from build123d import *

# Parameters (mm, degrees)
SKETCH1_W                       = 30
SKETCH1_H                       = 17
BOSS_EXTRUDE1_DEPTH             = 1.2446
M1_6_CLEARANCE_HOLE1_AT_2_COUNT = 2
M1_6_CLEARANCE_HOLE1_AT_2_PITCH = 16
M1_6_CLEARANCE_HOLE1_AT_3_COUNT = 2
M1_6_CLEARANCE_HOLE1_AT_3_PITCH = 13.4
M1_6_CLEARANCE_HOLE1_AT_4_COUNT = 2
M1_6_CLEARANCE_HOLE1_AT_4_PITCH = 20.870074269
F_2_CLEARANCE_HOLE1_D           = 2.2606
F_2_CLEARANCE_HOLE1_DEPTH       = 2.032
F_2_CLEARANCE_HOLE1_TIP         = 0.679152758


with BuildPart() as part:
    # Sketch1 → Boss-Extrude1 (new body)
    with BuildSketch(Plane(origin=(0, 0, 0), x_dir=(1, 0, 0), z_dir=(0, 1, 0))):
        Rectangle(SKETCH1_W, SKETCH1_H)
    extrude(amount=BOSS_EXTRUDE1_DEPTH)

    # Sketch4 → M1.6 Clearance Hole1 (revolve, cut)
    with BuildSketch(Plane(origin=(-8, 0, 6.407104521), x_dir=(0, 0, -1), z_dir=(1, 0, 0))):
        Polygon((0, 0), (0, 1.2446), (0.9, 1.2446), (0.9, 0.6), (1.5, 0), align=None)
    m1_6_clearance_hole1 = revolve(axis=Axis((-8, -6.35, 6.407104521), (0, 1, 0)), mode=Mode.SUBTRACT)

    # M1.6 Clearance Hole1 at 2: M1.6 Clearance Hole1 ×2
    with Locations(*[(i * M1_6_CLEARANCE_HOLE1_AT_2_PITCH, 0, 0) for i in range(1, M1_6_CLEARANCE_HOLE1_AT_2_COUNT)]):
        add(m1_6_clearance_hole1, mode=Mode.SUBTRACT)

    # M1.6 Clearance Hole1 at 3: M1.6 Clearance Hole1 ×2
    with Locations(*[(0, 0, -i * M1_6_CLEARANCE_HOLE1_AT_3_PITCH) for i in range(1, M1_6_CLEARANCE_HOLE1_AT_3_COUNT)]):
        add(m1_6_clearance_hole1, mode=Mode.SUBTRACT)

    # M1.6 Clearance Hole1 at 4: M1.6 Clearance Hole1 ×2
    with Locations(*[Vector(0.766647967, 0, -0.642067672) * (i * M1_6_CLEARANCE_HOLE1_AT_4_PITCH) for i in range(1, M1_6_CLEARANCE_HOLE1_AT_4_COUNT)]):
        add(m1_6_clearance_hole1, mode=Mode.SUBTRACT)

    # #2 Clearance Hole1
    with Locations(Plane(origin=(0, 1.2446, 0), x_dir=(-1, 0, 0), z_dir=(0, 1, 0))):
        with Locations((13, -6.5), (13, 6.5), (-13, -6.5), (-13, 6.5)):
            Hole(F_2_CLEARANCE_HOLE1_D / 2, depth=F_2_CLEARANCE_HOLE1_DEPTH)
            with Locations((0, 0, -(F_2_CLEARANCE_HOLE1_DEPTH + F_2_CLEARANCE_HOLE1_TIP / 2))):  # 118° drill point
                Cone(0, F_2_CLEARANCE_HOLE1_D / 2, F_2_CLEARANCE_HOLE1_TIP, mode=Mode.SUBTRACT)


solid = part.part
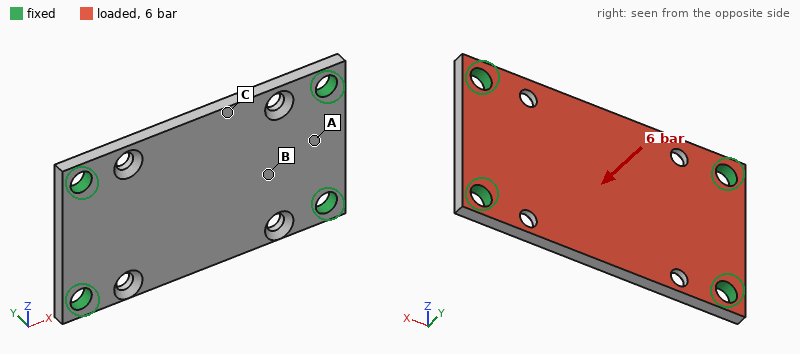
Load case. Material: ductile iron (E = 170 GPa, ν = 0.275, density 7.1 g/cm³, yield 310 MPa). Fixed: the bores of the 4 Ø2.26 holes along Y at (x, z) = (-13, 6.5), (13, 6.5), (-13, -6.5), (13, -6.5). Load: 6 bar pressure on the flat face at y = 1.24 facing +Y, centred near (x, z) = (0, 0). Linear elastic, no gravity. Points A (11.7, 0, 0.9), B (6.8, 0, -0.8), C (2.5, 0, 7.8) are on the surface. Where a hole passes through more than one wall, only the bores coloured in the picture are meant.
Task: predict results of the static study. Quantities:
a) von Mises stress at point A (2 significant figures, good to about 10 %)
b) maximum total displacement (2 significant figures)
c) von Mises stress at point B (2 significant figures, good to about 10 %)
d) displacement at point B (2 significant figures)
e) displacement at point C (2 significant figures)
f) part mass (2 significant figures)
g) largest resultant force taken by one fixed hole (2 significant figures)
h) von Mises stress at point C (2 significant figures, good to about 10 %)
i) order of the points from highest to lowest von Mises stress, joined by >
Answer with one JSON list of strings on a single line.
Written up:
["40 MPa", "26 µm", "19 MPa", "15 µm", "24 µm", "4.2 g", "73 N", "62 MPa", "C > A > B"]
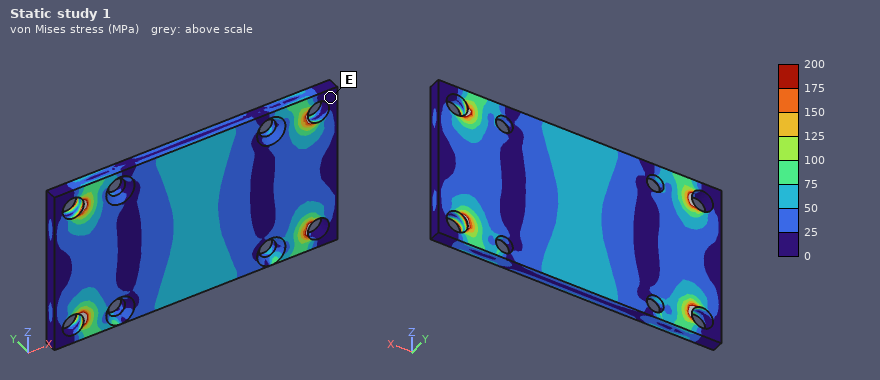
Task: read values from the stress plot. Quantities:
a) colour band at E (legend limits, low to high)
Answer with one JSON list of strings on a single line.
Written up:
["0 to 25 MPa"]
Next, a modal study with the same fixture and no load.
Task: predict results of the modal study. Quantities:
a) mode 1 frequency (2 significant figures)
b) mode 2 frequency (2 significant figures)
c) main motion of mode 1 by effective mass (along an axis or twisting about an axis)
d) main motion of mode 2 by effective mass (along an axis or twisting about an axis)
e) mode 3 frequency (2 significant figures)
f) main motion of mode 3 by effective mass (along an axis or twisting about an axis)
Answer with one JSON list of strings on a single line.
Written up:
["9200 Hz", "14 kHz", "along Y", "twisting about X", "24 kHz", "twisting about Z"]
